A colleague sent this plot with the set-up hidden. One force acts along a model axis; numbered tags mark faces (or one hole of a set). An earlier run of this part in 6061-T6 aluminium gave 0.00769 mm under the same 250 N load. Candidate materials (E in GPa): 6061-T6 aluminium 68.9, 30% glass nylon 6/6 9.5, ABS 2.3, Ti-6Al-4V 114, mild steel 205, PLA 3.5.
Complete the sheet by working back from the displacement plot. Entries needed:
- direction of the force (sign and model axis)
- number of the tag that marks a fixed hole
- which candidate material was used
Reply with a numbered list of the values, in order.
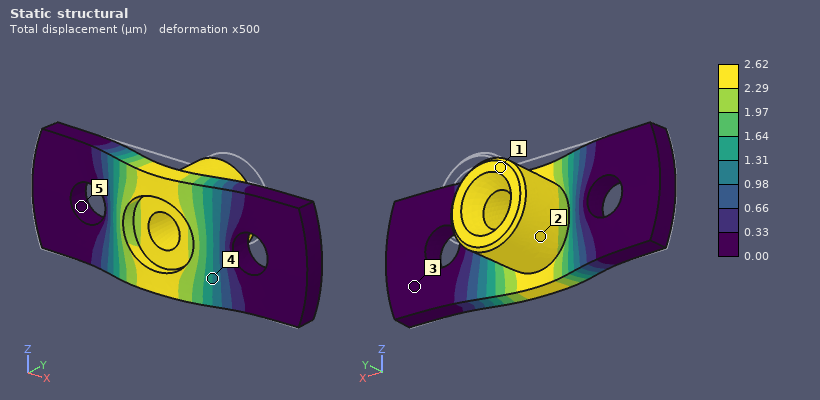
1. -Y
2. 5
3. mild steel
